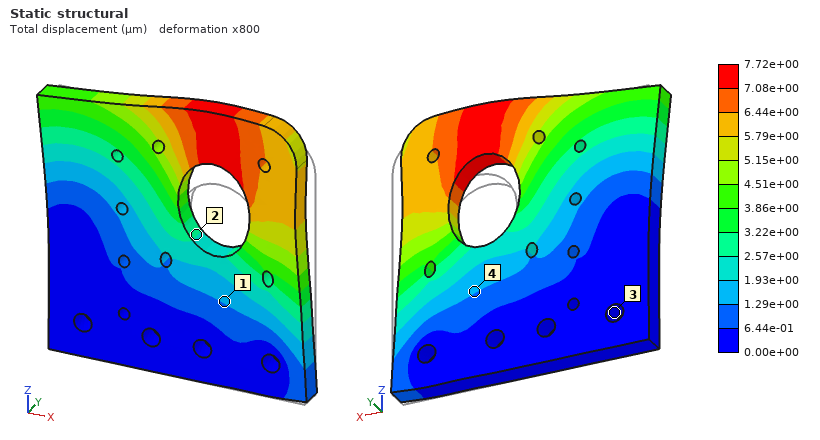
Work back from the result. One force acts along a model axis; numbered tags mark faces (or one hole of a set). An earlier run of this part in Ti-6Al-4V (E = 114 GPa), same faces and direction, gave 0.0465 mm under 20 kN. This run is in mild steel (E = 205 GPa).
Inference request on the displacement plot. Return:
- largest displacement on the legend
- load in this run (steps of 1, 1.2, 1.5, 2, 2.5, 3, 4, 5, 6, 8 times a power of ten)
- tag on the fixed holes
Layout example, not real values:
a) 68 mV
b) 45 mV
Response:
a) 7.72e+00 µm
b) 6 kN
c) 3
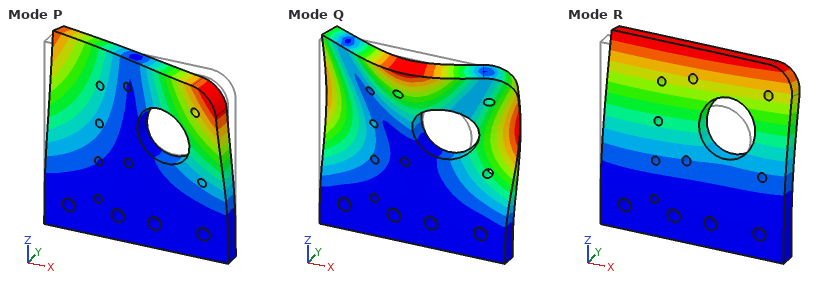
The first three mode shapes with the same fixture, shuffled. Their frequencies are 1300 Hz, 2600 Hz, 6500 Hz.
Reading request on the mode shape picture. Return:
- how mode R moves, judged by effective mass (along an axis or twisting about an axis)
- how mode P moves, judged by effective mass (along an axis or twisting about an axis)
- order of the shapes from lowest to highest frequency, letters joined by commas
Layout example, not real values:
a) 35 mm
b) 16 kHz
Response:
a) along Y
b) twisting about Z
c) R, P, Q
